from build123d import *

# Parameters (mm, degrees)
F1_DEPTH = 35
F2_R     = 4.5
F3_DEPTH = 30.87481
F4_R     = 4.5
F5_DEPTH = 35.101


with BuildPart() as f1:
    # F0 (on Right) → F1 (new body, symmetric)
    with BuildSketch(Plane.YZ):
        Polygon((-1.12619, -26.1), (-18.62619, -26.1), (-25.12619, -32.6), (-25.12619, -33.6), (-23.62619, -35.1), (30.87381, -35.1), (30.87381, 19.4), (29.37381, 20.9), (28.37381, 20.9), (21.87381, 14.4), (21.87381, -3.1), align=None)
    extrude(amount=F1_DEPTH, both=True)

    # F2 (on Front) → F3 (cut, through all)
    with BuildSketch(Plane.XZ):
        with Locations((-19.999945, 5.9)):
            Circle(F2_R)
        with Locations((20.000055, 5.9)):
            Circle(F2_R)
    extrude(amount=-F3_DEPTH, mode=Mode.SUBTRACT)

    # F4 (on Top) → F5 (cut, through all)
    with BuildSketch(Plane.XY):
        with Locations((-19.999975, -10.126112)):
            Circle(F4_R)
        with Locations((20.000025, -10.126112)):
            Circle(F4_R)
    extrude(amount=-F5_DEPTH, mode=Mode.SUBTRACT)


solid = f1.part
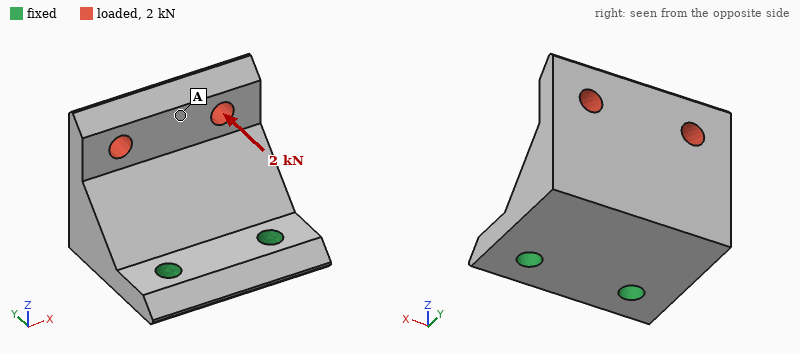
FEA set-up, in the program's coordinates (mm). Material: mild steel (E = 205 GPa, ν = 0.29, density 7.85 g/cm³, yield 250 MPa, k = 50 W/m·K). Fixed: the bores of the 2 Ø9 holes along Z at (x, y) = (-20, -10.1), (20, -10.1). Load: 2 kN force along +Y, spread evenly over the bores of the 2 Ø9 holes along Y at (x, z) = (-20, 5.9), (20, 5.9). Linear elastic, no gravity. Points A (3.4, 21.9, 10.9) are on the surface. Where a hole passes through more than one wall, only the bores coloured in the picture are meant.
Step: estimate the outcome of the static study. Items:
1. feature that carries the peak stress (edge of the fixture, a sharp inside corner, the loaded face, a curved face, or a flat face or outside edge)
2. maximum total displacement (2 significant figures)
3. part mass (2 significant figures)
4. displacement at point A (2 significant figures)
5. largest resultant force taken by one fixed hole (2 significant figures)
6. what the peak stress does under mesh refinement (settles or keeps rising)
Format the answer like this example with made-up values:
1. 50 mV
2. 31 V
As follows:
1. edge of the fixture
2. 78 µm
3. 610 g
4. 59 µm
5. 1.0 kN
6. keeps rising
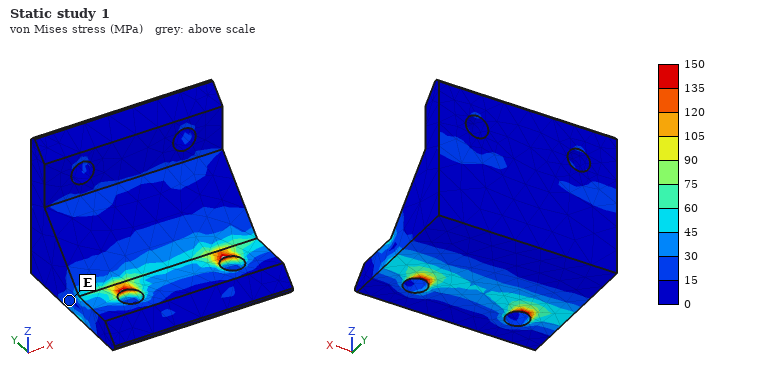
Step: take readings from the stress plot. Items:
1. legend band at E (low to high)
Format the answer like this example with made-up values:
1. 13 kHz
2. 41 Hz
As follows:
1. 15 to 30 MPa
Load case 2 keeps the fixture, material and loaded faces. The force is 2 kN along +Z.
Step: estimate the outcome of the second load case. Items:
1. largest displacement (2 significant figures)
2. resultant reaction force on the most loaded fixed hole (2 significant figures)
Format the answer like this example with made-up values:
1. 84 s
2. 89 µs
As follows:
1. 56 µm
2. 1.0 kN
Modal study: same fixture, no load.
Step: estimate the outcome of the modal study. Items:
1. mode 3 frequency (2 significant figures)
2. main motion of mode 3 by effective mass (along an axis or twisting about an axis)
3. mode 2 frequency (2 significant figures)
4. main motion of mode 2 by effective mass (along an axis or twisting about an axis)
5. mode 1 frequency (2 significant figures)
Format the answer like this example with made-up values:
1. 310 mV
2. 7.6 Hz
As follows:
1. 7600 Hz
2. along X
3. 4600 Hz
4. along X
5. 1800 Hz
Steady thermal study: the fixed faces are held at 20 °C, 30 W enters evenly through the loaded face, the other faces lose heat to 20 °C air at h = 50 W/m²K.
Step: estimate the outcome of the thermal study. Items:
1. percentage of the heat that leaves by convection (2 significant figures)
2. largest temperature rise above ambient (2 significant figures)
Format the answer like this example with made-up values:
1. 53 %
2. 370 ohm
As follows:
1. 38 %
2. 36 K
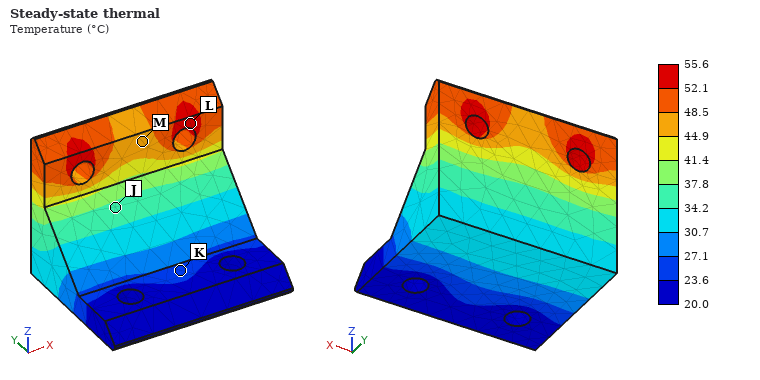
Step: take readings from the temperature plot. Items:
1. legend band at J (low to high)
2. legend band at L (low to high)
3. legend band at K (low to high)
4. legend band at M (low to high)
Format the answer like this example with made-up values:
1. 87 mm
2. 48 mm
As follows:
1. 34.2 to 37.8 °C
2. 52.1 to 55.6 °C
3. 23.6 to 27.1 °C
4. 44.9 to 48.5 °C
